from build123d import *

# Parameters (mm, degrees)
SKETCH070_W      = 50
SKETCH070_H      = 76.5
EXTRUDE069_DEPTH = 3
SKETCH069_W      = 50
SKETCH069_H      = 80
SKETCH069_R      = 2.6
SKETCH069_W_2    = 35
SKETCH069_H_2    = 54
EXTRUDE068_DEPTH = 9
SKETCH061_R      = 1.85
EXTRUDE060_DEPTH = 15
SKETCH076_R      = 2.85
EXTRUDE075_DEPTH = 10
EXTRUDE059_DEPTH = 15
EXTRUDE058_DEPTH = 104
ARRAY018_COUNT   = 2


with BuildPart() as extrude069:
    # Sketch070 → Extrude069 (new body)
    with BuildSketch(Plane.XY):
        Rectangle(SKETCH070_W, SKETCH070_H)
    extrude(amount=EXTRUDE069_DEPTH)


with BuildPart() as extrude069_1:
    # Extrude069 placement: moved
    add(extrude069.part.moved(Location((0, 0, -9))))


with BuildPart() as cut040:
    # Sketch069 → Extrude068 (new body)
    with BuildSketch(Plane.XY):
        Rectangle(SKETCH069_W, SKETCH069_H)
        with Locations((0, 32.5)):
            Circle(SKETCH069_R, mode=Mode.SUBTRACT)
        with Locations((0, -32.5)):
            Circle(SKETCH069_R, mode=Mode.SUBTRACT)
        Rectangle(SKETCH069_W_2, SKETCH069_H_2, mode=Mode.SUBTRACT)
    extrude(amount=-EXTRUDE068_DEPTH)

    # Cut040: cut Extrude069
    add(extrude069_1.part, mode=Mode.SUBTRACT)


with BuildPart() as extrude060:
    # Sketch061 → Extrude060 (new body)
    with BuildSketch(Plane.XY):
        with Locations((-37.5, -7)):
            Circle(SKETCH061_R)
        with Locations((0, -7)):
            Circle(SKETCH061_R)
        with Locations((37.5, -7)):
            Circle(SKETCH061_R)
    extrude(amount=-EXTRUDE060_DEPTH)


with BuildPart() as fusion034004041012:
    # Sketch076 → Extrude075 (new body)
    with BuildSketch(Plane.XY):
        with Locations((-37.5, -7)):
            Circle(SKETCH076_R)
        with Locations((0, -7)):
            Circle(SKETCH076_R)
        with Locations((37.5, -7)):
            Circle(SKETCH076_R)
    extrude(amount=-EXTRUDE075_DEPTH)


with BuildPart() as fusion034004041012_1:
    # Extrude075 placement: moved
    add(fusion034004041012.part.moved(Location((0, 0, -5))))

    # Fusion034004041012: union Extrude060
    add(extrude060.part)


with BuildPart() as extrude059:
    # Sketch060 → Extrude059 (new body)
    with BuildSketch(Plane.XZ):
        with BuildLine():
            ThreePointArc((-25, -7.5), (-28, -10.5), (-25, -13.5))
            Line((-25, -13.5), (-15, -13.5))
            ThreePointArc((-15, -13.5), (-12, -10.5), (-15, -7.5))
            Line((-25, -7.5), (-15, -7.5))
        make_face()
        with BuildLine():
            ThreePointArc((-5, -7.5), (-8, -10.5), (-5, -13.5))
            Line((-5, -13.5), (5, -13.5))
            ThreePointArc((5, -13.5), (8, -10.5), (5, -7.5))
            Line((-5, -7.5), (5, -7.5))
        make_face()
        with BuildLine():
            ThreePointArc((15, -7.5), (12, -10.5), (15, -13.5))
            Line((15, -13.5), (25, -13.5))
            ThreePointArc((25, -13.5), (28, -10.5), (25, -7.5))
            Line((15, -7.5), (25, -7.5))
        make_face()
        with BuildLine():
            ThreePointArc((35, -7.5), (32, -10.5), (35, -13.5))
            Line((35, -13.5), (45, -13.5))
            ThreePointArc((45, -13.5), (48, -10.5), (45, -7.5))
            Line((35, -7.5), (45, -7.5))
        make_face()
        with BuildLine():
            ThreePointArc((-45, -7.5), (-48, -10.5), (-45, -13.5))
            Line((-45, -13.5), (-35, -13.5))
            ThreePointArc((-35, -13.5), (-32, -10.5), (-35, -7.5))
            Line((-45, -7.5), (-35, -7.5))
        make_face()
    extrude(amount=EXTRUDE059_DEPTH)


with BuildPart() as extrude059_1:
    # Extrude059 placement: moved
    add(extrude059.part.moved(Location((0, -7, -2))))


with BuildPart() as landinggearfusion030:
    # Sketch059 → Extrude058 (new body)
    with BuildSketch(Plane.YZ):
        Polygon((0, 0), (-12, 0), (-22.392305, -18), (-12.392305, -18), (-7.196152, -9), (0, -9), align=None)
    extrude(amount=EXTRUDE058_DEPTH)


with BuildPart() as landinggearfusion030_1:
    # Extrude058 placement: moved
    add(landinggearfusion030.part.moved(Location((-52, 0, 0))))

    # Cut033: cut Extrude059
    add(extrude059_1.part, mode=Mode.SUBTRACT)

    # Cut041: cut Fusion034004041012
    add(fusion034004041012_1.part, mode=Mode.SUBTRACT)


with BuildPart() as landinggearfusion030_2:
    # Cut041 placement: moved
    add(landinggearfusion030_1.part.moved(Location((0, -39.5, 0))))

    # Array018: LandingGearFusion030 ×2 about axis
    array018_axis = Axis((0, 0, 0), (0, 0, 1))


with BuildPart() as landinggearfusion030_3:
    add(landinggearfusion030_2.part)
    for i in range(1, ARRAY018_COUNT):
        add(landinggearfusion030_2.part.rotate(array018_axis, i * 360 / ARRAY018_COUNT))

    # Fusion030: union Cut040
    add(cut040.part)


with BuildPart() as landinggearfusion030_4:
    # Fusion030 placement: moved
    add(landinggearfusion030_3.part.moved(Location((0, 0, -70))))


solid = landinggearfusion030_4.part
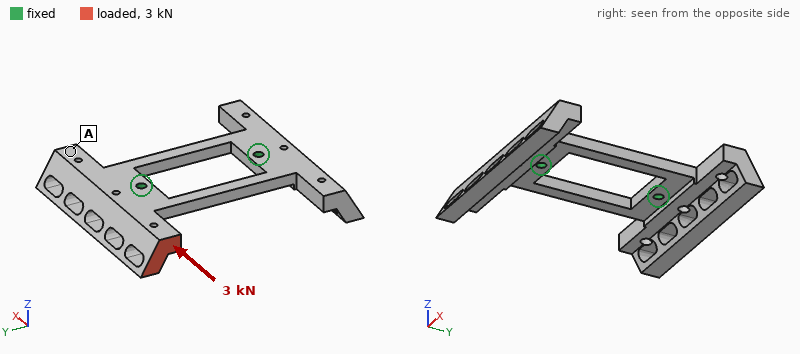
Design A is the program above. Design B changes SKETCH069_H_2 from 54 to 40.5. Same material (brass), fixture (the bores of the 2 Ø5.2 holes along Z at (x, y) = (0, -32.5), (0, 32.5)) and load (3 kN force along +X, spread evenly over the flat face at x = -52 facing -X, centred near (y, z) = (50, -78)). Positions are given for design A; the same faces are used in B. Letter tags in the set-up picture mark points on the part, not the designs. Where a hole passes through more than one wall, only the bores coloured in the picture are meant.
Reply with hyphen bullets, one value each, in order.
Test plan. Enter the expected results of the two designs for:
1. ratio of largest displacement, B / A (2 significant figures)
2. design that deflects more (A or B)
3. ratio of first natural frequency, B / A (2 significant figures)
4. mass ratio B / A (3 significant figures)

- 0.88
- A
- 1.1
- 1.06
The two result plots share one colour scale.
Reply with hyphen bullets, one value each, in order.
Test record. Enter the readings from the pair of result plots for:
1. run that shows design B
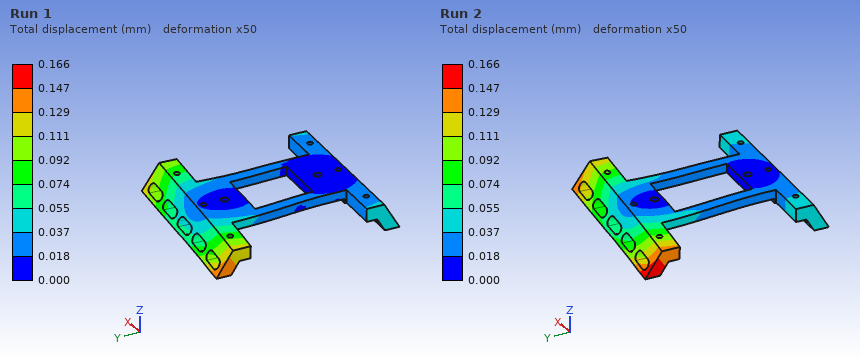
- Run 1
